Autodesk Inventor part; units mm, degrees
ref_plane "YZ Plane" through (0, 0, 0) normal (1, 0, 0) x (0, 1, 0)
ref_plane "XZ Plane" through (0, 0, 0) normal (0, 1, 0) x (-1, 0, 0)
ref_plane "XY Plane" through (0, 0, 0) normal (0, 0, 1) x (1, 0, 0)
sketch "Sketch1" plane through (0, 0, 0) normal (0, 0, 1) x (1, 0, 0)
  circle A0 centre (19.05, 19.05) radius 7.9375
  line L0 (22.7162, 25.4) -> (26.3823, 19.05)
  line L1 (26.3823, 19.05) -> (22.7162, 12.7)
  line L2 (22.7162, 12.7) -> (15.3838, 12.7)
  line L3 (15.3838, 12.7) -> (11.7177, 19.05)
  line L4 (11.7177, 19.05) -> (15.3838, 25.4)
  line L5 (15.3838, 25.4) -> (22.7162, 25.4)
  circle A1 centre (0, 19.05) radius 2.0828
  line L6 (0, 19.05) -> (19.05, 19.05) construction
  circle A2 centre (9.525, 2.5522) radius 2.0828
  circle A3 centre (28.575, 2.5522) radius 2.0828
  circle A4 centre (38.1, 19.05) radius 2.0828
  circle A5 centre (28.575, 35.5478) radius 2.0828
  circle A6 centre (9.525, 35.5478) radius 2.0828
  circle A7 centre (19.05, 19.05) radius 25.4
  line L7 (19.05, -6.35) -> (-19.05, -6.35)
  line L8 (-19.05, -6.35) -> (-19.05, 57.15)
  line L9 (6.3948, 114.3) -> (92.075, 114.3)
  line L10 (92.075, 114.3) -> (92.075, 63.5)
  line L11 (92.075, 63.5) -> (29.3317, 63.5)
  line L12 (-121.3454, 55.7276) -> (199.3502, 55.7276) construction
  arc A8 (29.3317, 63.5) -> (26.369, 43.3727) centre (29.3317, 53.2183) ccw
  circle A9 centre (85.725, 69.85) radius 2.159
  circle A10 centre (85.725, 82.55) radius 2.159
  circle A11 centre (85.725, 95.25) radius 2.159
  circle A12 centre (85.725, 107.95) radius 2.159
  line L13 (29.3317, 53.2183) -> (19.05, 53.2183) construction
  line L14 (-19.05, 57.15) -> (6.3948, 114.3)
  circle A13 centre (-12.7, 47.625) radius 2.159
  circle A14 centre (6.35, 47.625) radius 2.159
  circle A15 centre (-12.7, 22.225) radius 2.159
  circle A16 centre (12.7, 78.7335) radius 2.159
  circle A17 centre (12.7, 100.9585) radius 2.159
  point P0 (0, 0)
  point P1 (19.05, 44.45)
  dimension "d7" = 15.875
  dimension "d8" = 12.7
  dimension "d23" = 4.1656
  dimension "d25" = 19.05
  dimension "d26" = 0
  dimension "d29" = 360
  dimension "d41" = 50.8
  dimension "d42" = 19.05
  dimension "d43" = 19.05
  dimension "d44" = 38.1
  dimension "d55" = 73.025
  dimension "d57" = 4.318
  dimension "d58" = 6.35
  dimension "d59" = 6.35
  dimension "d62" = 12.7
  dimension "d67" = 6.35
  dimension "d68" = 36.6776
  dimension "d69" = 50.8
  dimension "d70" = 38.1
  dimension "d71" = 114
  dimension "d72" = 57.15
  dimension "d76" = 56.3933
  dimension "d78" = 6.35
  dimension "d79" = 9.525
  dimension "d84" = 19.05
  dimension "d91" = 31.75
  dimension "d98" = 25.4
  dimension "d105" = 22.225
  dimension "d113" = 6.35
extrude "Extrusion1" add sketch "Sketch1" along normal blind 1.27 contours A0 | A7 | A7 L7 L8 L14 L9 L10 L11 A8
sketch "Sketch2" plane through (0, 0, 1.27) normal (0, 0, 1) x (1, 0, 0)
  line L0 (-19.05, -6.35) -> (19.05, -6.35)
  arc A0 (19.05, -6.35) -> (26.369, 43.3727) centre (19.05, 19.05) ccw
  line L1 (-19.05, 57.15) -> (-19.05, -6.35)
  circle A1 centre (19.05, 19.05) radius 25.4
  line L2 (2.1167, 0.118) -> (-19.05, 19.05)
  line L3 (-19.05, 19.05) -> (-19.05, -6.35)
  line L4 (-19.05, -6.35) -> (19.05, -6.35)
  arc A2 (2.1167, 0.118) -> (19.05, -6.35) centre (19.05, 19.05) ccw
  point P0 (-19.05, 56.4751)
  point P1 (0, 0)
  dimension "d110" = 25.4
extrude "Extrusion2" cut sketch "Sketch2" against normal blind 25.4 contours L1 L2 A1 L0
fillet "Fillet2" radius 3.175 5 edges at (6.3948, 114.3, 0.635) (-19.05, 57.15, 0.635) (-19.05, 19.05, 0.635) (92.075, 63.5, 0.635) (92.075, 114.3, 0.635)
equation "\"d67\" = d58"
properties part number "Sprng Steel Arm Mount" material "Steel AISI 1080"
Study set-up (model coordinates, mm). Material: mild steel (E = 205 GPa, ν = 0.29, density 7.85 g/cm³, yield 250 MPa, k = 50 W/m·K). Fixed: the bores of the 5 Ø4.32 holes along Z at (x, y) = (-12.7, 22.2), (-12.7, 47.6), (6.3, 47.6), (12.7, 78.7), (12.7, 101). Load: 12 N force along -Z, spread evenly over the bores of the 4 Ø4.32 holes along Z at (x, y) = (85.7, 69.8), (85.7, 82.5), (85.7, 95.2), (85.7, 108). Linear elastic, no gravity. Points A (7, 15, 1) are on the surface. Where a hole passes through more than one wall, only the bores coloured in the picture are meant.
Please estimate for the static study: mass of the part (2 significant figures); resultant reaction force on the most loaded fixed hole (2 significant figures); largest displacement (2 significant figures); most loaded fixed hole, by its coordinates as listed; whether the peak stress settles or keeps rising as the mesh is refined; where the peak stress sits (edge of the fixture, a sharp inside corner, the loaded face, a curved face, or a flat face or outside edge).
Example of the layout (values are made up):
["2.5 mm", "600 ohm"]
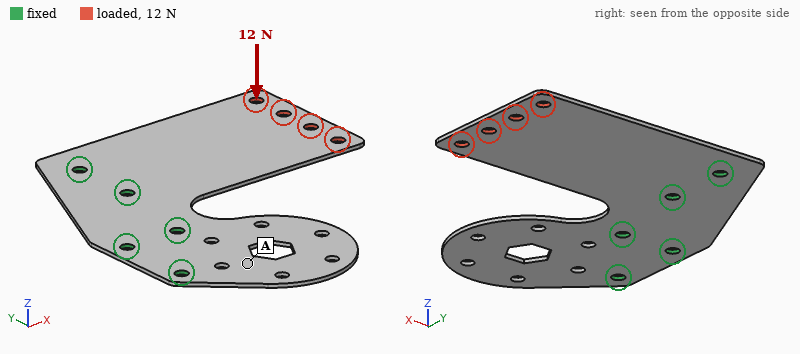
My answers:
["79 g", "11 N", "0.92 mm", "(12.7, 78.7)", "keeps rising", "edge of the fixture"]
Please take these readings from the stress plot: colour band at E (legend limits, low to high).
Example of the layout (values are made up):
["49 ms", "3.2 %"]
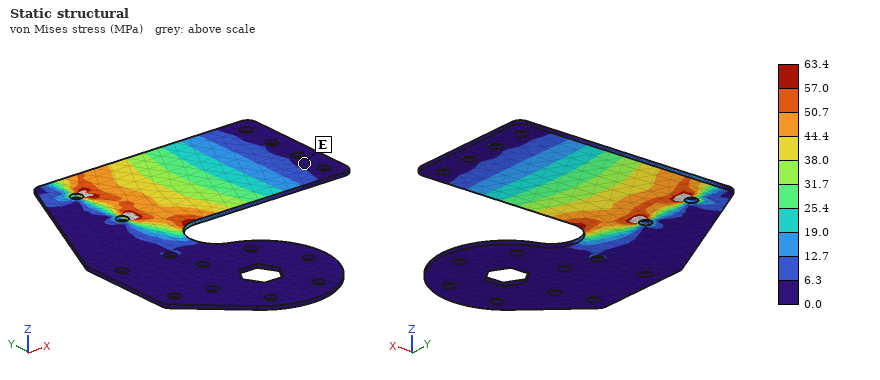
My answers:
["0.0 to 6.3 MPa"]
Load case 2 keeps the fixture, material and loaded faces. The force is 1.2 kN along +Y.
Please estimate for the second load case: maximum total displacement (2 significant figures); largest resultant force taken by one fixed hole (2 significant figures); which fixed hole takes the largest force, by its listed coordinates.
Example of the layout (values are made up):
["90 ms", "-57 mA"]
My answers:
["0.10 mm", "2.6 kN", "(12.7, 101)"]
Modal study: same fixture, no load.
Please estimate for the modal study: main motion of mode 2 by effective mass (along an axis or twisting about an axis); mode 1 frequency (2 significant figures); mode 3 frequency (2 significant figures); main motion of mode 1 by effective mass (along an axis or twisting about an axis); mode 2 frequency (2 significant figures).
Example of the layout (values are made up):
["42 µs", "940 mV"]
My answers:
["along Z", "180 Hz", "600 Hz", "along Z", "460 Hz"]
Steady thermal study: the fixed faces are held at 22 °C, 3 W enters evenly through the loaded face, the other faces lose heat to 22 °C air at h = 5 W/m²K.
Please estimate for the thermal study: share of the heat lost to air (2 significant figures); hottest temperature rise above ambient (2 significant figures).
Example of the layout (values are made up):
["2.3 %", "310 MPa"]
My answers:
["37 %", "53 K"]
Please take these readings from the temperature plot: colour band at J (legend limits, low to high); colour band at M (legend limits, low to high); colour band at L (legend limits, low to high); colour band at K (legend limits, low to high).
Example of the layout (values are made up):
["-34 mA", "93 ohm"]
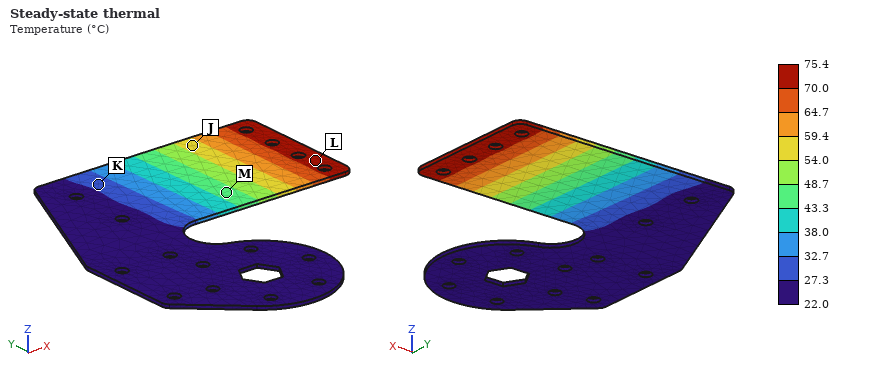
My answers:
["54.0 to 59.4 °C", "43.3 to 48.7 °C", "70.0 to 75.4 °C", "27.3 to 32.7 °C"]
